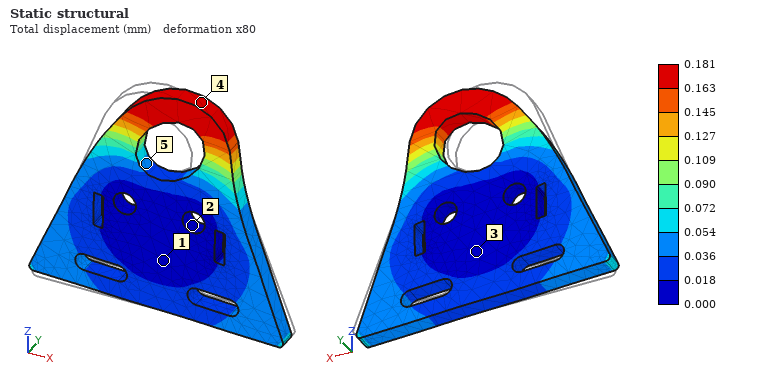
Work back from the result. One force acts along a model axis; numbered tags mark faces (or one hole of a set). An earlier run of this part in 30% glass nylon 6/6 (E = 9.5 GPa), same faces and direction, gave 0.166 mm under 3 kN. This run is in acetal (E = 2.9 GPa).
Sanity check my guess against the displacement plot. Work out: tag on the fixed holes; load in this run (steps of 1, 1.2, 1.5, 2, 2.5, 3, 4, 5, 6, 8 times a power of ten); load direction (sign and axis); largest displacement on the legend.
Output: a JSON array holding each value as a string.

["2", "1 kN", "+X", "0.181 mm"]
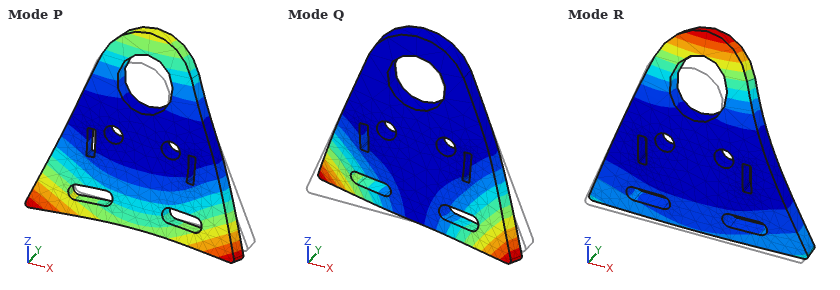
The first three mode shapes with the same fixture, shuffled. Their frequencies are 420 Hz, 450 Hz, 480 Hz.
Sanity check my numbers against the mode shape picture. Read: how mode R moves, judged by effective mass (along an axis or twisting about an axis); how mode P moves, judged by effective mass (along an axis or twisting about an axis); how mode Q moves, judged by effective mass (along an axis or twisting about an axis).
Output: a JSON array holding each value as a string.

["along Y", "along Y", "twisting about Z"]
